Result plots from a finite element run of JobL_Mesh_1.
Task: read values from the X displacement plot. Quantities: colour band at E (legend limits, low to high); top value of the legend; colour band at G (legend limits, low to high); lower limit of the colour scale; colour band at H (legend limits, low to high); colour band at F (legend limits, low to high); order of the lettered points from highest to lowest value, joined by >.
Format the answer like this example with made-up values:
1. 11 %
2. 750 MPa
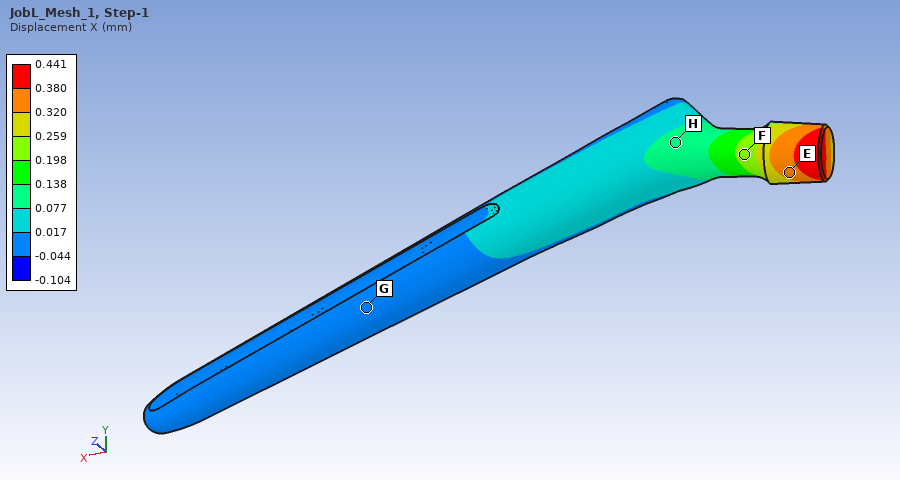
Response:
1. 0.320 to 0.380 mm
2. 0.441 mm
3. -0.044 to 0.017 mm
4. -0.104 mm
5. 0.077 to 0.138 mm
6. 0.198 to 0.259 mm
7. E > F > H > G
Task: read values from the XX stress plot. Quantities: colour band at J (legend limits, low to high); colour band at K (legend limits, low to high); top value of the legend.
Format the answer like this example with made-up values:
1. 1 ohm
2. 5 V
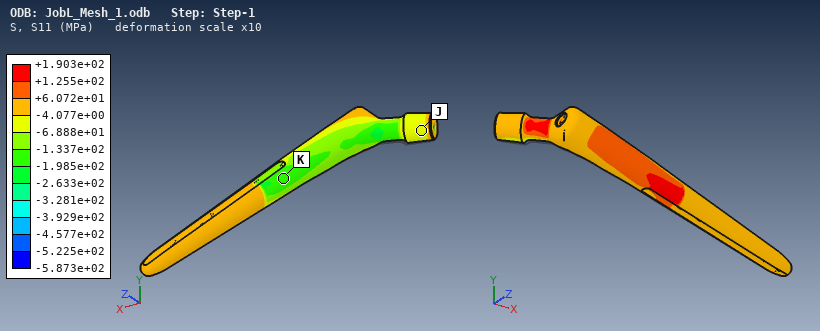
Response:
1. -6.888e+01 to -4.077e+00 MPa
2. -1.985e+02 to -1.337e+02 MPa
3. +1.903e+02 MPa
